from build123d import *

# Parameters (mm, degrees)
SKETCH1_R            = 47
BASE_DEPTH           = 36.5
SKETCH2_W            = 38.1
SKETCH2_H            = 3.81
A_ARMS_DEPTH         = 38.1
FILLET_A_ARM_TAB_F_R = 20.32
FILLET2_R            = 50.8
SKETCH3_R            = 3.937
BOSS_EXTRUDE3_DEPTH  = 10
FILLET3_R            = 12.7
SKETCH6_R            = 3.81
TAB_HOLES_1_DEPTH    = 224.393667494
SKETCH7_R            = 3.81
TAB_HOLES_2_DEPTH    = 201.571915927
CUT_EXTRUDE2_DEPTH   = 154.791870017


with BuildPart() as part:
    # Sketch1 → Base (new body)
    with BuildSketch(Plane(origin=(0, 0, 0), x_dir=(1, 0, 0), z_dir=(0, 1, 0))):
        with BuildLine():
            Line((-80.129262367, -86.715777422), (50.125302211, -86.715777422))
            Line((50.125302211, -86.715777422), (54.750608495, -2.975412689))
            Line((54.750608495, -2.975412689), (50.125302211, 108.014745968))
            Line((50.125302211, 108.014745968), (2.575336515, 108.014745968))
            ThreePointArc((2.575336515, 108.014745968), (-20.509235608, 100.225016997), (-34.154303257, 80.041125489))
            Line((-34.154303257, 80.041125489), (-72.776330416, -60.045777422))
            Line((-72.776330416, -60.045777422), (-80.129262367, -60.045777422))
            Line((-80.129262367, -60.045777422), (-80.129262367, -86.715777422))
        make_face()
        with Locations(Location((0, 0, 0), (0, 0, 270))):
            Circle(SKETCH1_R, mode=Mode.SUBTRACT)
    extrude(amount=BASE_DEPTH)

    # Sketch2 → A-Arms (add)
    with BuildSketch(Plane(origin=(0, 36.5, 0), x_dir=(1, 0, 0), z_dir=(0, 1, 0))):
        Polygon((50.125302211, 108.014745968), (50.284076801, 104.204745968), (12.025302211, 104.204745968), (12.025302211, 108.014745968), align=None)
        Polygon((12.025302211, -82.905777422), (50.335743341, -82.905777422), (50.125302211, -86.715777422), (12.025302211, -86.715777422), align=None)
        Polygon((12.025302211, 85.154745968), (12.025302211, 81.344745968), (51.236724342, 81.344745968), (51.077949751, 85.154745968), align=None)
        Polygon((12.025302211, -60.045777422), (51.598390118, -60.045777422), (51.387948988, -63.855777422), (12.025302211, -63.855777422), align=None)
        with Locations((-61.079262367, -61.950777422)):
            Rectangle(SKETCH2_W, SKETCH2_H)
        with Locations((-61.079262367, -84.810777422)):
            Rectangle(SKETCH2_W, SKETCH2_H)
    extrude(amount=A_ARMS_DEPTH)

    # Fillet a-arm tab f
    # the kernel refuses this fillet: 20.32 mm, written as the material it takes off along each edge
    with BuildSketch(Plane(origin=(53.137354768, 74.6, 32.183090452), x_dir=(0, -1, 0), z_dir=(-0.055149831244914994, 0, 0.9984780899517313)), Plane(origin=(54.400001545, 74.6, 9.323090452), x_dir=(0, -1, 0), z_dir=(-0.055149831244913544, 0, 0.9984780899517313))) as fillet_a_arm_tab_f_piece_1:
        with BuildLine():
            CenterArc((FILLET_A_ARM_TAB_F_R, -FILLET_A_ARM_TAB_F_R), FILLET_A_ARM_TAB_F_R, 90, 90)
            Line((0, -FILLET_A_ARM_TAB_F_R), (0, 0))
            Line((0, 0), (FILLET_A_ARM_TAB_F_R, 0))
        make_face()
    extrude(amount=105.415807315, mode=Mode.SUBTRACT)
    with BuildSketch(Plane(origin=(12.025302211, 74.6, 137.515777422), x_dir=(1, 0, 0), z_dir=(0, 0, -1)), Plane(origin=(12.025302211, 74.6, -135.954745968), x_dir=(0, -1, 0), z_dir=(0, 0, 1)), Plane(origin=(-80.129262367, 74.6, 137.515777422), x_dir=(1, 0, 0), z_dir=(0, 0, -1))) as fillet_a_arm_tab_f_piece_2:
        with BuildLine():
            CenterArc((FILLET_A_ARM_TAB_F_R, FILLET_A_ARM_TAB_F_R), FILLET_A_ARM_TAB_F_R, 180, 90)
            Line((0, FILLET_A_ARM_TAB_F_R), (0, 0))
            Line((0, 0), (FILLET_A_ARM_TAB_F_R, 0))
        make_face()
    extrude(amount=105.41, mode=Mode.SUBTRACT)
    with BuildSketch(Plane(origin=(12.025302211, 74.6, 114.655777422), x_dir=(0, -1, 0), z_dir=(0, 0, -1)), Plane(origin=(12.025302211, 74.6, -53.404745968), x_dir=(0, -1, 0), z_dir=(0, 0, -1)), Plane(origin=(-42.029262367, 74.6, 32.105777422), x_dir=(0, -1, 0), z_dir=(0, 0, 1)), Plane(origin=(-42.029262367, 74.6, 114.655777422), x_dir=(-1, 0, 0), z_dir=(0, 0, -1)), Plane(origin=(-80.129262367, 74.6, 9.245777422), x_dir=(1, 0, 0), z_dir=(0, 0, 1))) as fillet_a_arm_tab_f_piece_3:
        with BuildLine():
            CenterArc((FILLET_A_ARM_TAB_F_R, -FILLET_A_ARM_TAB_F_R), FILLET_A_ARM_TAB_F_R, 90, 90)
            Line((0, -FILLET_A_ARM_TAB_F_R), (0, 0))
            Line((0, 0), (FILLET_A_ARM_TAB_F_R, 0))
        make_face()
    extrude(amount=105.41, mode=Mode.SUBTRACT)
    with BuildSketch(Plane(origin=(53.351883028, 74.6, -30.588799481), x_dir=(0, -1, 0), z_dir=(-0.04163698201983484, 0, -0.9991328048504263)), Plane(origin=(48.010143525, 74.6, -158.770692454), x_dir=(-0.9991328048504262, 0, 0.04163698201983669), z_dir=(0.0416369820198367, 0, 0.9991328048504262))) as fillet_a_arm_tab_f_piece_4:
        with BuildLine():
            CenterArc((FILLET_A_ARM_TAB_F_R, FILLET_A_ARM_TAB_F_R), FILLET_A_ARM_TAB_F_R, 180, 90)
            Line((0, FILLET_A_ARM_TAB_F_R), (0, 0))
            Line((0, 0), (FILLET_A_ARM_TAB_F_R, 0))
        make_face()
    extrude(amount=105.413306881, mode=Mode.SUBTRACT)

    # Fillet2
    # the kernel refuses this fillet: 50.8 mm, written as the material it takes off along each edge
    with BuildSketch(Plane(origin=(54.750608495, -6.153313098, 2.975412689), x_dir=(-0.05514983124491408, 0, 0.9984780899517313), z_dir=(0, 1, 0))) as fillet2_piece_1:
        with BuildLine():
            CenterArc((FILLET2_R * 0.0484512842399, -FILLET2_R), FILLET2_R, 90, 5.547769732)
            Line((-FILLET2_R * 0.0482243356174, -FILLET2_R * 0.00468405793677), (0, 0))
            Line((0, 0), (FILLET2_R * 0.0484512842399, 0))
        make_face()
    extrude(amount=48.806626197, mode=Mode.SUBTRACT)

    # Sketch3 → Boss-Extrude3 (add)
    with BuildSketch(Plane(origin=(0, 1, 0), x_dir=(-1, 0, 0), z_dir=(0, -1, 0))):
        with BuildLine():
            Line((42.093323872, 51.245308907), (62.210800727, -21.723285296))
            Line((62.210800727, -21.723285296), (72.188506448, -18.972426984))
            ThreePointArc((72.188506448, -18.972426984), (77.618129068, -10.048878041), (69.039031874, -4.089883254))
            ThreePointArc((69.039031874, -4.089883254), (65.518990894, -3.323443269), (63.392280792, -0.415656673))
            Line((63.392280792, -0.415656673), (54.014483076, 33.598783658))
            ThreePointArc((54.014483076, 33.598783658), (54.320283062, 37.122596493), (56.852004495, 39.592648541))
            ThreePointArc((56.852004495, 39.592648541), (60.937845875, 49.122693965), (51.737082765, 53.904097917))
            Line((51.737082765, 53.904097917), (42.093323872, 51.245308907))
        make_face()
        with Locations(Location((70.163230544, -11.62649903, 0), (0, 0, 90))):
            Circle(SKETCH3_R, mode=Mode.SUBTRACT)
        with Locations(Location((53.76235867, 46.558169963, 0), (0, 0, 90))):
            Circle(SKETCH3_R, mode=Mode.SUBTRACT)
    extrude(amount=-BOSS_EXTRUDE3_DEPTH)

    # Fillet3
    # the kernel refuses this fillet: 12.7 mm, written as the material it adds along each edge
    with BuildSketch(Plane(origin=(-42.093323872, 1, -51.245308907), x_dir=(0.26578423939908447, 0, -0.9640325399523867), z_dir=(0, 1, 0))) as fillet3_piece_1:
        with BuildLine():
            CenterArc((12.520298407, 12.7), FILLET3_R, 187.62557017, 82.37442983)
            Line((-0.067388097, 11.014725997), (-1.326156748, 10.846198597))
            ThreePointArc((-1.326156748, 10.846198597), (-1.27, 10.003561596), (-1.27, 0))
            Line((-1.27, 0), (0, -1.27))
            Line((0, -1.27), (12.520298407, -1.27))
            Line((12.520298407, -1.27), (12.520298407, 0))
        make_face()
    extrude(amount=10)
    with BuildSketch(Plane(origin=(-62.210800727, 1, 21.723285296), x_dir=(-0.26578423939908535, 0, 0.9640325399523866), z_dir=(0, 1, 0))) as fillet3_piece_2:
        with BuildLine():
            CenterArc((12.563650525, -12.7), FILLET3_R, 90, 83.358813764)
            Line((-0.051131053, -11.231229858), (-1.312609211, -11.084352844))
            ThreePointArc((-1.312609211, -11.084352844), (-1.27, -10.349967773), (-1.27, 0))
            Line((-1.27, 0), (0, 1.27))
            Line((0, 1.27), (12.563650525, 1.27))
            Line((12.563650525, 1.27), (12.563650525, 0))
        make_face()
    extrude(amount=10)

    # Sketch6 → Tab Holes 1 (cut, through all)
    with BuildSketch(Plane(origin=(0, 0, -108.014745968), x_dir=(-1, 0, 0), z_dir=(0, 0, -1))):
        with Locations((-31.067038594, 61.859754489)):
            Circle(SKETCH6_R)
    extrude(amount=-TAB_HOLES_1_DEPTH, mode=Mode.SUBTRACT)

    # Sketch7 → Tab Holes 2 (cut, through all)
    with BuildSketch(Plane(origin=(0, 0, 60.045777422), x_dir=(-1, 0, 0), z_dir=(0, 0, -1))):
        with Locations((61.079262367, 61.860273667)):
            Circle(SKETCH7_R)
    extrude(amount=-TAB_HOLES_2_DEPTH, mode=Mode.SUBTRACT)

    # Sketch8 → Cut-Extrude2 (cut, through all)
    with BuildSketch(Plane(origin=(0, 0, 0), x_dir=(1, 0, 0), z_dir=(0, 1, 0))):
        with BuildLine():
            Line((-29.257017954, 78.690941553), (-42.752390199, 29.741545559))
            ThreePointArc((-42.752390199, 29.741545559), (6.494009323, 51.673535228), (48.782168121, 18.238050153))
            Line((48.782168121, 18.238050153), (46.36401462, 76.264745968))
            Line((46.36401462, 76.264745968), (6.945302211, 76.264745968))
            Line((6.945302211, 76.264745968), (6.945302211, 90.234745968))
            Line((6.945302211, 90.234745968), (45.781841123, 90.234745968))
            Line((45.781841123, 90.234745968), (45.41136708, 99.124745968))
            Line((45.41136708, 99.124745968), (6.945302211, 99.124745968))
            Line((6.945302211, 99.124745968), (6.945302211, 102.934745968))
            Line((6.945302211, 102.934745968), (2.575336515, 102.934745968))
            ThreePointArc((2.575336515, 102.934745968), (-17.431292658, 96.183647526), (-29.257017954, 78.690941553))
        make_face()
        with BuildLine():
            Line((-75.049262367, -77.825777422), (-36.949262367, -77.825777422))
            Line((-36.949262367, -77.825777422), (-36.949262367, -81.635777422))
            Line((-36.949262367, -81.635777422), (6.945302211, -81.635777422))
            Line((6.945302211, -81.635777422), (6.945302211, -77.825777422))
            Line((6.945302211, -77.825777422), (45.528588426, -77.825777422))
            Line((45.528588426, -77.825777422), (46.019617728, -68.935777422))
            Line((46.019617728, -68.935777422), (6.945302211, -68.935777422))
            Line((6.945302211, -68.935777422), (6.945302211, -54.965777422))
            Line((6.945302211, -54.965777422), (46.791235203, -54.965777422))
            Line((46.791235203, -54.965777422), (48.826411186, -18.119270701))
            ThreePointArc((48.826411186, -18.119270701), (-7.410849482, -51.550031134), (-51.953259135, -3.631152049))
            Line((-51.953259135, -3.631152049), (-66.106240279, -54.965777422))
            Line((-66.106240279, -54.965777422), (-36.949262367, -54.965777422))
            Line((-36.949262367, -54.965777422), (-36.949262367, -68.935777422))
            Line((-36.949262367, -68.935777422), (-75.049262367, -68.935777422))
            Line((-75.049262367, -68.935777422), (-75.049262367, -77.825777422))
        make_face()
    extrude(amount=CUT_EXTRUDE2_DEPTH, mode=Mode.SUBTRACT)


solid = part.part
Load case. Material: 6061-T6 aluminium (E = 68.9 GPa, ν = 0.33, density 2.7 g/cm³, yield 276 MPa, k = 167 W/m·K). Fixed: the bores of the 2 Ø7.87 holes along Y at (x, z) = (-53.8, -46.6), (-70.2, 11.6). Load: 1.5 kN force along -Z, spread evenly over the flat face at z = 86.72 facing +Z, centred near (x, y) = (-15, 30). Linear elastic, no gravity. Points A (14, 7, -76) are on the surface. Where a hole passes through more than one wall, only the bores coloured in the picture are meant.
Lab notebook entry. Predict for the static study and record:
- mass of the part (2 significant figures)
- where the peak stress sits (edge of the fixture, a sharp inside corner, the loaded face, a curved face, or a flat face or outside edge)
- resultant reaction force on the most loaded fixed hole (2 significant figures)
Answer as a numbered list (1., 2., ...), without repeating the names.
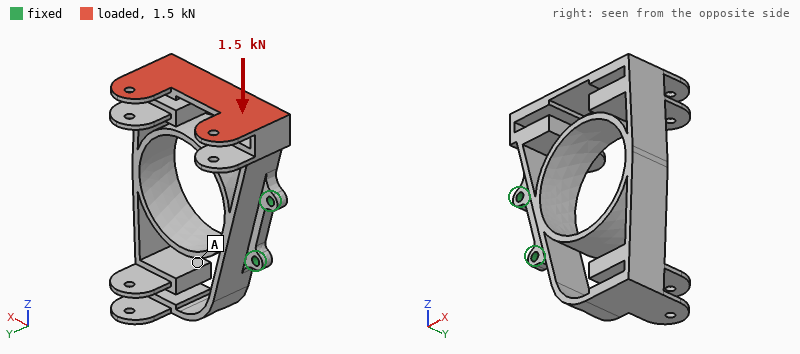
1. 730 g
2. a flat face or outside edge
3. 1.5 kN
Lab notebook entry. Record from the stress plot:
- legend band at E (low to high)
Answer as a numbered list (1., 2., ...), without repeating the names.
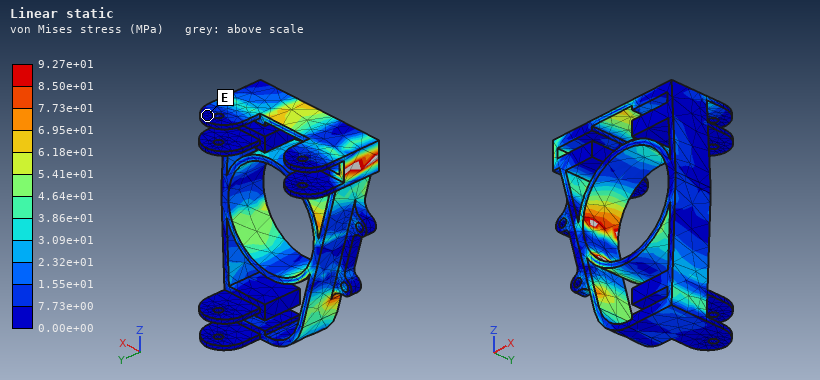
1. 0.00e+00 to 7.73e+00 MPa
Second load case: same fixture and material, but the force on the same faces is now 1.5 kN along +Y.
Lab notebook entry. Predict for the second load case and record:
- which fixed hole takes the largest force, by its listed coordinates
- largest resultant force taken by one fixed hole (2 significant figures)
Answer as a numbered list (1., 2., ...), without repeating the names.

1. (-70.2, 11.6)
2. 2.7 kN
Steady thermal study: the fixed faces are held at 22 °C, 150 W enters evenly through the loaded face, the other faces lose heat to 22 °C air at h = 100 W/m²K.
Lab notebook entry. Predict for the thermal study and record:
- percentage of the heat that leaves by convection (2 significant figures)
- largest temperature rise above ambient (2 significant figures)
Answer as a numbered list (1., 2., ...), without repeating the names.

1. 91 %
2. 71 K
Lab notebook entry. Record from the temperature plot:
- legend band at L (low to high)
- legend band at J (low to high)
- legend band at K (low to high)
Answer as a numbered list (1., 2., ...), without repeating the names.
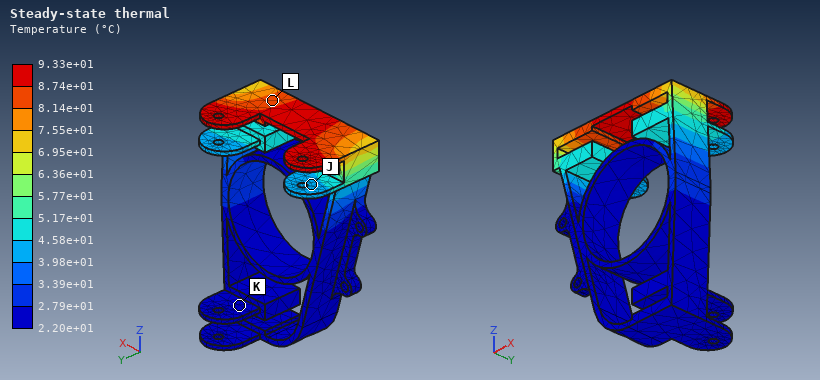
1. 8.14e+01 to 8.74e+01 °C
2. 3.98e+01 to 4.58e+01 °C
3. 2.20e+01 to 2.79e+01 °C
